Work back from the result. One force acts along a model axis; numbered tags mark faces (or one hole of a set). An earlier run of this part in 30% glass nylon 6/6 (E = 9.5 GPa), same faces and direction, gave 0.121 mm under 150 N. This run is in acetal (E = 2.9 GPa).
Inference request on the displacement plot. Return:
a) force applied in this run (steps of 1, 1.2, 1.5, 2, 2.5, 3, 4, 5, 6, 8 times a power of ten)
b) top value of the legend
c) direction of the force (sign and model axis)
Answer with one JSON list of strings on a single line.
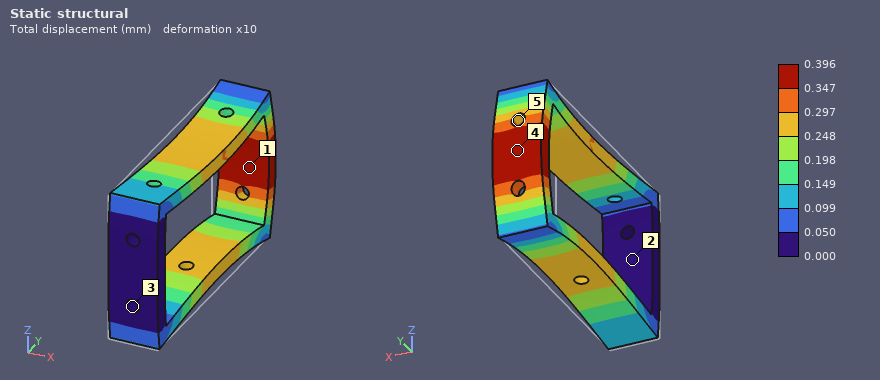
["150 N", "0.396 mm", "+Y"]
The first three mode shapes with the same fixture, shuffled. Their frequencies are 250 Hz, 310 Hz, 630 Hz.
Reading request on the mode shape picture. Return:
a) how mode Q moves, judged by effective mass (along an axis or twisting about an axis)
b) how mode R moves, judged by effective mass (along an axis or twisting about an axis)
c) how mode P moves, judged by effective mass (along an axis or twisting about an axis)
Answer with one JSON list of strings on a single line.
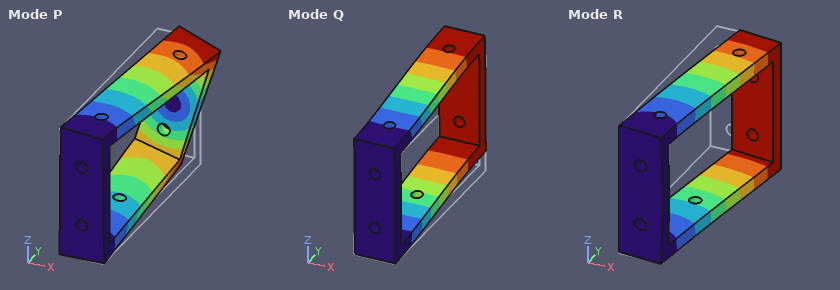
["along Z", "along X", "twisting about Y"]
